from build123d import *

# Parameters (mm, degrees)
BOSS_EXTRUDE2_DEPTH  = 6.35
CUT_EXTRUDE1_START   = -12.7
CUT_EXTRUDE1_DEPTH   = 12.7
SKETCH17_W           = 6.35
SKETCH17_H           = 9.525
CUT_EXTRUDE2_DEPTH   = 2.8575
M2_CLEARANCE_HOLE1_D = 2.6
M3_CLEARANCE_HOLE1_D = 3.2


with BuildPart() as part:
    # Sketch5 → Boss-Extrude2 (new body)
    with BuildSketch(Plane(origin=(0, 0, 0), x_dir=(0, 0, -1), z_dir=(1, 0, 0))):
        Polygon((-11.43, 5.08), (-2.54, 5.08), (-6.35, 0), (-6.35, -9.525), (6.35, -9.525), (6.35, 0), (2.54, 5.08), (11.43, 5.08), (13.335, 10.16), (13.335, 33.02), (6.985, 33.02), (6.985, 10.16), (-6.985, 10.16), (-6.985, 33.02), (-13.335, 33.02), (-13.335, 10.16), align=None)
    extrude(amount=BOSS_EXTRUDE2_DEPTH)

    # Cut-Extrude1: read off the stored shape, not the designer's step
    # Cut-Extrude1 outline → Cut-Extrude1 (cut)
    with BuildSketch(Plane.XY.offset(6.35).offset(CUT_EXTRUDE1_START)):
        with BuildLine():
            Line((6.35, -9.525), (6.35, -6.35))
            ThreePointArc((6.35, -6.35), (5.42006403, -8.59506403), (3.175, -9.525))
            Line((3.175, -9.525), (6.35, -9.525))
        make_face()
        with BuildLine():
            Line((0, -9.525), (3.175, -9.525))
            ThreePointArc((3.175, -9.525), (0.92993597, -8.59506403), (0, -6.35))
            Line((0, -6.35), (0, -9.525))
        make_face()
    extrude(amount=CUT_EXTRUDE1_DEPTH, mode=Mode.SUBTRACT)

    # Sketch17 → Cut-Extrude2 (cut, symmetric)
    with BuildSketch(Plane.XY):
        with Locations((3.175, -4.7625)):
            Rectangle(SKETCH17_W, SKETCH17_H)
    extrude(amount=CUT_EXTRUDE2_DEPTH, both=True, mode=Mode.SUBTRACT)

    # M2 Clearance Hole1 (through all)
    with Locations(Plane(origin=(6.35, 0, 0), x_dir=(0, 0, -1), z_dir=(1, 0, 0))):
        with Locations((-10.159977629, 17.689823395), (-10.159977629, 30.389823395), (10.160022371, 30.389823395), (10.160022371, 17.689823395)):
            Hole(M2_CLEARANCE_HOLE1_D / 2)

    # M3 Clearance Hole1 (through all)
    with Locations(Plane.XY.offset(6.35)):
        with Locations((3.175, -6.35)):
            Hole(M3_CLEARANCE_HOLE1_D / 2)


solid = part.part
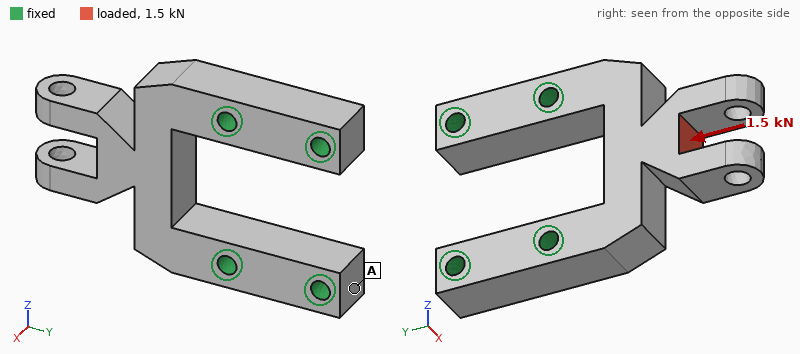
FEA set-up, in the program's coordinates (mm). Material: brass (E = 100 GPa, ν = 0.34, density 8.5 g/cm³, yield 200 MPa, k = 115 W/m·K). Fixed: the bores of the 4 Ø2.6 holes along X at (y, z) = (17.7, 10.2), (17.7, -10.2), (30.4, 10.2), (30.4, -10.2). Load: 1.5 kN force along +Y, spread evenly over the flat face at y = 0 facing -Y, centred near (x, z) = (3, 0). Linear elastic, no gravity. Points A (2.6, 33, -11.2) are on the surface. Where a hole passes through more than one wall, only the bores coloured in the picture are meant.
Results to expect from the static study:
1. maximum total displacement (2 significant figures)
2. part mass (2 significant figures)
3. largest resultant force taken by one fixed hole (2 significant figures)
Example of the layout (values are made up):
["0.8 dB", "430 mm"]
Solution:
["14 µm", "27 g", "830 N"]
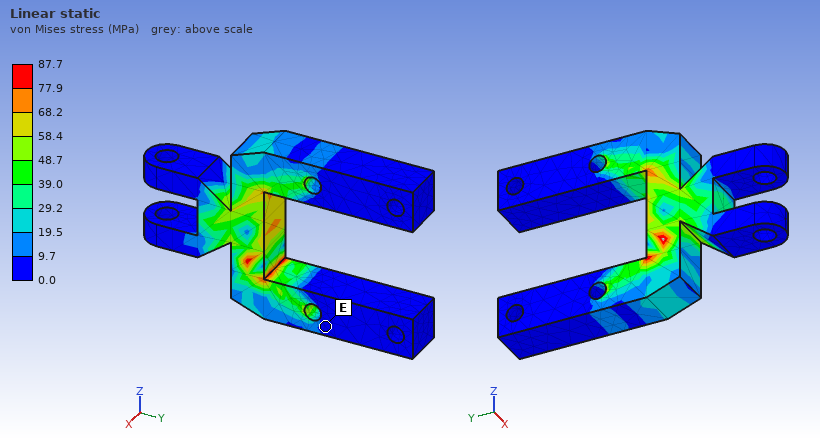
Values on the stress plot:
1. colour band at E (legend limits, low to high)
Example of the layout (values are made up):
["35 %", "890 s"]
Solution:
["0.0 to 9.7 MPa"]
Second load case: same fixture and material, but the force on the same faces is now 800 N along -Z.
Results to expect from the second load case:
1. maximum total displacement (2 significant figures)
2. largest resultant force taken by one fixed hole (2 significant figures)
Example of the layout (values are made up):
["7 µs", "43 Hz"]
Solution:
["46 µm", "670 N"]
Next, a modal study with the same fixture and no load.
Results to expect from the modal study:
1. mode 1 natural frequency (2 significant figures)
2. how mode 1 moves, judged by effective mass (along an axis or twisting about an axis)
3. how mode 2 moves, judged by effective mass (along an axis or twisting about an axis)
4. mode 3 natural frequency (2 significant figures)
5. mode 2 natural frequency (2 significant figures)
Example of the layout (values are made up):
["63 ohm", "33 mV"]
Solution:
["5100 Hz", "along X", "along Z", "13 kHz", "8400 Hz"]
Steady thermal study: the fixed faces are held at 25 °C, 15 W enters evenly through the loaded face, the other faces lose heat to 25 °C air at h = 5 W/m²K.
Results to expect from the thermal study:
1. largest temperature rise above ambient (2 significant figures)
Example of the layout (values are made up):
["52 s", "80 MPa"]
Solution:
["48 K"]
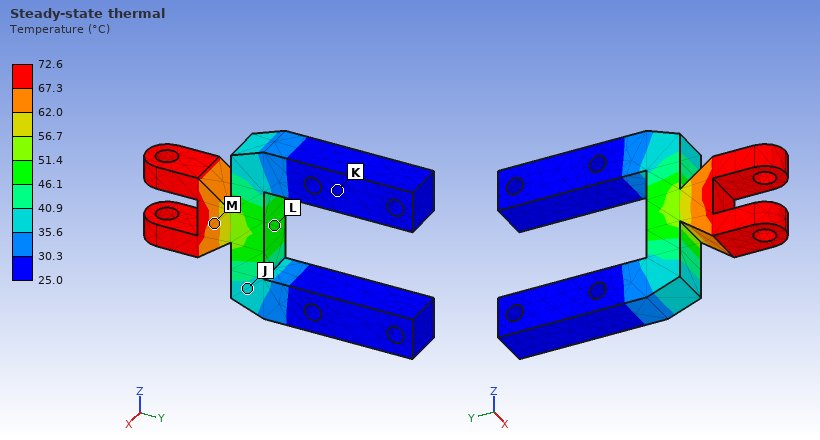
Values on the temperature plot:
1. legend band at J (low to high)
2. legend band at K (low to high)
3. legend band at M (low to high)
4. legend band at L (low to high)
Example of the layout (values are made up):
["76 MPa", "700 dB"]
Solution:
["35.6 to 40.9 °C", "25.0 to 30.3 °C", "62.0 to 67.3 °C", "46.1 to 51.4 °C"]
